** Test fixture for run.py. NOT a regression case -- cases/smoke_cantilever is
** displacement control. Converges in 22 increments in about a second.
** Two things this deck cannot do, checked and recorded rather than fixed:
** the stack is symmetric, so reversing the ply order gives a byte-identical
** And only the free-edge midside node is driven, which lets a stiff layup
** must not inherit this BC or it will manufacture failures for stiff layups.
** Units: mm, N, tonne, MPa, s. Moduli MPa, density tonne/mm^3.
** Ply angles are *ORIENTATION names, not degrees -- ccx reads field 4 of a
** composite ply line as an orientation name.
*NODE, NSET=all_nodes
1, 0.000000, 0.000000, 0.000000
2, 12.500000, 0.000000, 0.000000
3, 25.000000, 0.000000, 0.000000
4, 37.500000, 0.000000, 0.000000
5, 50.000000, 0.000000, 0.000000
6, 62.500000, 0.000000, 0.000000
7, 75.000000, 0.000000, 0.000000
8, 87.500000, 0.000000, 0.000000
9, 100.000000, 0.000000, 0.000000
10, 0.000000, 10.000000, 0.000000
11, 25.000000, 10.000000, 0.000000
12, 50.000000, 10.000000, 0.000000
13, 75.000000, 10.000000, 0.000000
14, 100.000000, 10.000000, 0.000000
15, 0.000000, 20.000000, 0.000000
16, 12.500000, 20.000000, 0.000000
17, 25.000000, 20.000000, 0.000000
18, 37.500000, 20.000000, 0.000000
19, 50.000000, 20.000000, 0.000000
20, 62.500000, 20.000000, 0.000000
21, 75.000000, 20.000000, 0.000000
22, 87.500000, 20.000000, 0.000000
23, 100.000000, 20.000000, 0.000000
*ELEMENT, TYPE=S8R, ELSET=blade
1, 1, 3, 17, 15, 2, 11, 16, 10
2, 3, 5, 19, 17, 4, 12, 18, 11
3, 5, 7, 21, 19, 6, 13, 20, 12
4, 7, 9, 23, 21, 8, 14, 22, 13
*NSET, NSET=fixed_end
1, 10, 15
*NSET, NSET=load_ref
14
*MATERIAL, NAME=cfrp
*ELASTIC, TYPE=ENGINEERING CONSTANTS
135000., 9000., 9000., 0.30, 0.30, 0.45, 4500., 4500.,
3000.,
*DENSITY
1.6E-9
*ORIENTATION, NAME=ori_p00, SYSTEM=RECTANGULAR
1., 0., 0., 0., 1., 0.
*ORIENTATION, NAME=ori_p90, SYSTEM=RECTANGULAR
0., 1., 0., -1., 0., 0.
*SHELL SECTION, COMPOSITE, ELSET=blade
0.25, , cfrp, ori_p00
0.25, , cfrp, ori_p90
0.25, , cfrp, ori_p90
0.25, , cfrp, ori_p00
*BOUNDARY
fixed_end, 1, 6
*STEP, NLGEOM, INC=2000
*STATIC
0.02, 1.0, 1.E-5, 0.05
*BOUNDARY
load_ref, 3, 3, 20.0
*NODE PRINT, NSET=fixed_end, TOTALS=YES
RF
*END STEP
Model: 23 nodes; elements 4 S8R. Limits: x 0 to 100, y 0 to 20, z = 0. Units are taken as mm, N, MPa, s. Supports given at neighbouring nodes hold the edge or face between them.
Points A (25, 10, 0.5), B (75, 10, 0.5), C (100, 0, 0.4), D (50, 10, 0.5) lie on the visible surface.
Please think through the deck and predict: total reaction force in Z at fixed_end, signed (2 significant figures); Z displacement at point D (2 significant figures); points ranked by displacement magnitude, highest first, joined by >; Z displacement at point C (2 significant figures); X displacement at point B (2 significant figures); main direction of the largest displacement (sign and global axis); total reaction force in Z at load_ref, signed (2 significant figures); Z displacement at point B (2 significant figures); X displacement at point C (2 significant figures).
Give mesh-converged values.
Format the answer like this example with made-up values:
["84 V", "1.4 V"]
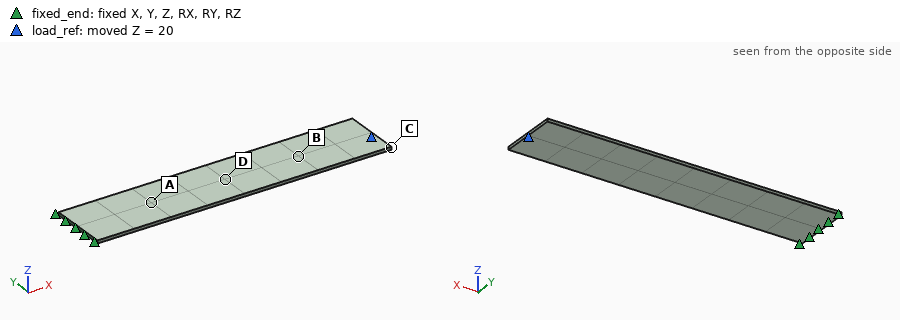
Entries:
["-12 N", "6.3 mm", "C > B > D > A", "20 mm", "-1.5 mm", "+Z", "12 N", "13 mm", "-2.5 mm"]
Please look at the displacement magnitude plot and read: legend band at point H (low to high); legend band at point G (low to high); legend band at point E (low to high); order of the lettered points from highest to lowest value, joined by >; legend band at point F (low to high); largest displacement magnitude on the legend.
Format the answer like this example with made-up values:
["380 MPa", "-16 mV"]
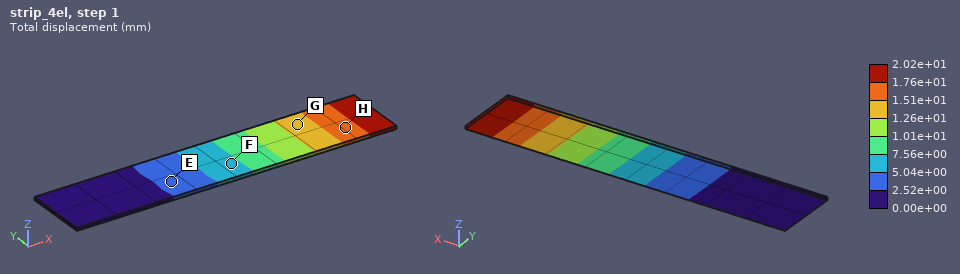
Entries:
["1.51e+01 to 1.76e+01 mm", "1.26e+01 to 1.51e+01 mm", "2.52e+00 to 5.04e+00 mm", "H > G > F > E", "5.04e+00 to 7.56e+00 mm", "2.02e+01 mm"]
